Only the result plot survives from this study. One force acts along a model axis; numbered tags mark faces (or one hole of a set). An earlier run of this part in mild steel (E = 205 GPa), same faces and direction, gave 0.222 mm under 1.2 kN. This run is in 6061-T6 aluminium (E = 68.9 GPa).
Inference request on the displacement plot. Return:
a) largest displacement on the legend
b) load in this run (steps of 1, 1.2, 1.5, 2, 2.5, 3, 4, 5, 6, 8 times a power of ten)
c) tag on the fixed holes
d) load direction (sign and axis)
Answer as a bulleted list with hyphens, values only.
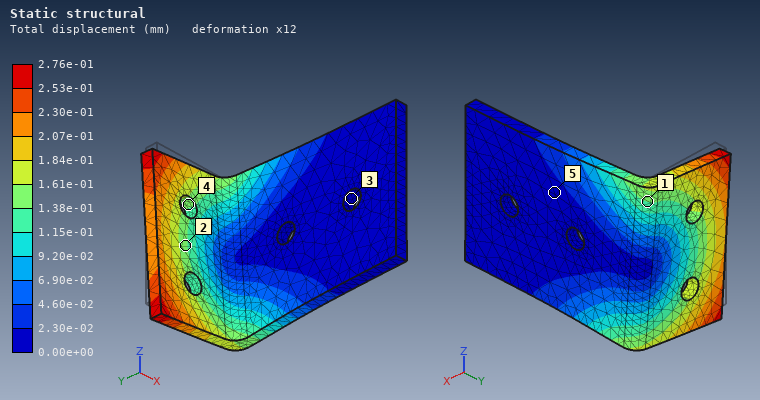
- 2.76e-01 mm
- 500 N
- 3
- -Z
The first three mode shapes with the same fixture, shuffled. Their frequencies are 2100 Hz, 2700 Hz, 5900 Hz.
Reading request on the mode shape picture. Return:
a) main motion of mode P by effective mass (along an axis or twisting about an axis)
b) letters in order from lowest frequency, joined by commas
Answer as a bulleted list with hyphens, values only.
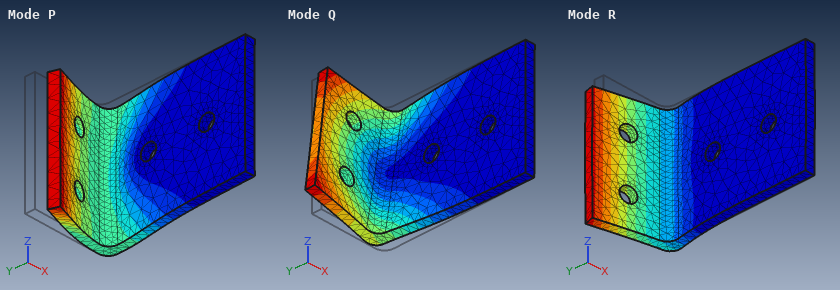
- along X
- R, Q, P
